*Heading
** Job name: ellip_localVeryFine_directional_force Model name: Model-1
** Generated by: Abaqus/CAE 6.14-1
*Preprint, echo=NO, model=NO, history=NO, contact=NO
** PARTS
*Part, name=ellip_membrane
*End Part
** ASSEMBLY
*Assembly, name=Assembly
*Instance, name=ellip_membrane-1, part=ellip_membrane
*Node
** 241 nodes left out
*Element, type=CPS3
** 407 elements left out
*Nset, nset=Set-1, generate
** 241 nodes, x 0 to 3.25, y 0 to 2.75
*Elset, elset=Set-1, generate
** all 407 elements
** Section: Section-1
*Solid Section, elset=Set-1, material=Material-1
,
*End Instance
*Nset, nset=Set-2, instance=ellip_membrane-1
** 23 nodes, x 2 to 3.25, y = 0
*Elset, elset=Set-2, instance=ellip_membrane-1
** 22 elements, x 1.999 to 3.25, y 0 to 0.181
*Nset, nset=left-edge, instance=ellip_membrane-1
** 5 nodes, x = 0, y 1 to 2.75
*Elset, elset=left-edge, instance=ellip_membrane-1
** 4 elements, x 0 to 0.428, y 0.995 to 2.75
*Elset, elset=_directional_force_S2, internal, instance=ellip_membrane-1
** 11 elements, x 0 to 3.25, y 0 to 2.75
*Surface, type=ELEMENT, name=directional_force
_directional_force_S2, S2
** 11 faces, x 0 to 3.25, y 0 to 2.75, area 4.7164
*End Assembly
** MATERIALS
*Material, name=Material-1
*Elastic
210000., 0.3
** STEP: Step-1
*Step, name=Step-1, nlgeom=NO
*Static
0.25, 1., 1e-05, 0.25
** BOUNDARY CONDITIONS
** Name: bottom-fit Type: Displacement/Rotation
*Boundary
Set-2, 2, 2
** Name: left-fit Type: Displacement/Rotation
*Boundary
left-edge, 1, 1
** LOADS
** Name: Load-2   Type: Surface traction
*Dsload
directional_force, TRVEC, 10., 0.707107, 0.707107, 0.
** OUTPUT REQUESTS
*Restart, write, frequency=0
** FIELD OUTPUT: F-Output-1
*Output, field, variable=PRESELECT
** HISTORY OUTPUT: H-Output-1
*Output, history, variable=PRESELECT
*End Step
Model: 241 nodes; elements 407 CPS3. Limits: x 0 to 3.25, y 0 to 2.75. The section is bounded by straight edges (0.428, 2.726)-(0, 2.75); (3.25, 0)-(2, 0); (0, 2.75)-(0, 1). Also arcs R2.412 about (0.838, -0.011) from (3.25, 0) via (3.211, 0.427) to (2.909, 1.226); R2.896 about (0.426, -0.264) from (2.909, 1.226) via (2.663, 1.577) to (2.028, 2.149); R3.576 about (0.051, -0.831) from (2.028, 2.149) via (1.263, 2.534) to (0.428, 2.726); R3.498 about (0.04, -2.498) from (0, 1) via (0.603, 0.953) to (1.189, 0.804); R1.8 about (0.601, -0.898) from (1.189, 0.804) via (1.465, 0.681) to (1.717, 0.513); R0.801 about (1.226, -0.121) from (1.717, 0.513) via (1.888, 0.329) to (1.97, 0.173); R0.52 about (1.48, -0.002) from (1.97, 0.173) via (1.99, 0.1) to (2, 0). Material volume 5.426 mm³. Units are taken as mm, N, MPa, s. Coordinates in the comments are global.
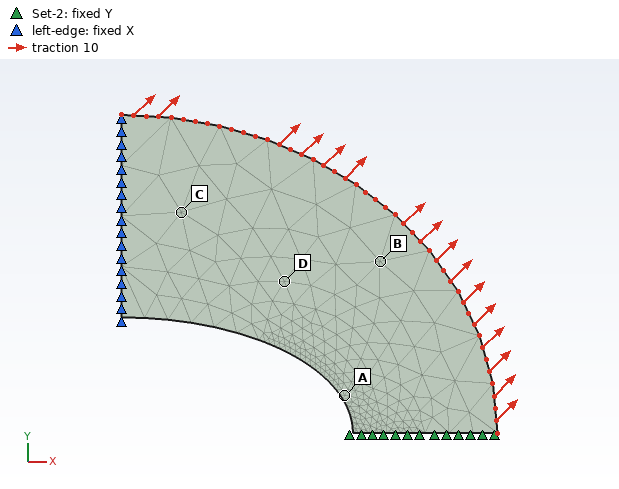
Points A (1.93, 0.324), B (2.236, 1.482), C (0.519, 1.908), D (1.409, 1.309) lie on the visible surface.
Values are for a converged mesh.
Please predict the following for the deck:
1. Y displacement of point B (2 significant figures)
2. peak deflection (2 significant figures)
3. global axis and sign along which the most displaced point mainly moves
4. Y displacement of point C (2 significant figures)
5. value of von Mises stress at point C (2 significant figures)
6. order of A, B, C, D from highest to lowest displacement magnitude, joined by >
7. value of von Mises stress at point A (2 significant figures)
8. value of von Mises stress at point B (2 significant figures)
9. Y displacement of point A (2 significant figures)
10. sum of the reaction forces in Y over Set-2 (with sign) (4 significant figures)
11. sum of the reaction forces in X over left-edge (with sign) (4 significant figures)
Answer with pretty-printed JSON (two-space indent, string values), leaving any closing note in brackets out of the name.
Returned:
{
  "Y displacement of point B": "1.6e-04 mm",
  "peak deflection": "4.7e-04 mm",
  "global axis and sign along which the most displaced point mainly moves": "+Y",
  "Y displacement of point C": "4.5e-04 mm",
  "value of von Mises stress at point C": "18 MPa",
  "order of A, B, C, D from highest to lowest displacement magnitude, joined by >": "C > D > B > A",
  "value of von Mises stress at point A": "50 MPa",
  "value of von Mises stress at point B": "13 MPa",
  "Y displacement of point A": "1.1e-04 mm",
  "sum of the reaction forces in Y over Set-2 (with sign)": "-33.35 N",
  "sum of the reaction forces in X over left-edge (with sign)": "-33.35 N"
}
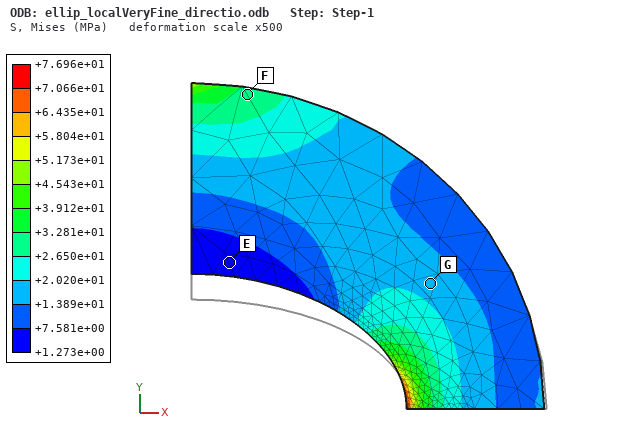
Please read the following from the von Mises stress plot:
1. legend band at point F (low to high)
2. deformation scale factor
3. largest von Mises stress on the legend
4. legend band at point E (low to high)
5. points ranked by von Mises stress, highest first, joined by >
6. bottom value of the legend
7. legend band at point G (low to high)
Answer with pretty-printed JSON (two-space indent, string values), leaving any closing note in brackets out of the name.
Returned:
{
  "legend band at point F": "+2.650e+01 to +3.281e+01 MPa",
  "deformation scale factor": "500",
  "largest von Mises stress on the legend": "+7.696e+01 MPa",
  "legend band at point E": "+1.273e+00 to +7.581e+00 MPa",
  "points ranked by von Mises stress, highest first, joined by >": "F > G > E",
  "bottom value of the legend": "+1.273e+00 MPa",
  "legend band at point G": "+1.389e+01 to +2.020e+01 MPa"
}
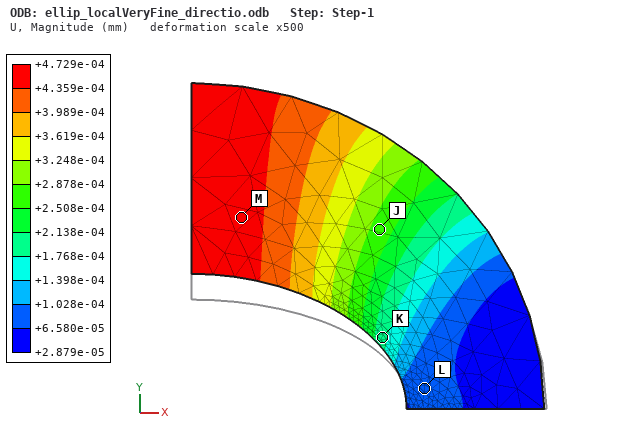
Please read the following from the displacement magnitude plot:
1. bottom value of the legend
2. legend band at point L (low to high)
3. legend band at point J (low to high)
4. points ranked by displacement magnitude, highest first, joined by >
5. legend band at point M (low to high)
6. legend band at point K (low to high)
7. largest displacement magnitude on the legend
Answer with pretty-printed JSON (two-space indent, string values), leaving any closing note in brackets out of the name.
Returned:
{
  "bottom value of the legend": "+2.879e-05 mm",
  "legend band at point L": "+6.580e-05 to +1.028e-04 mm",
  "legend band at point J": "+2.508e-04 to +2.878e-04 mm",
  "points ranked by displacement magnitude, highest first, joined by >": "M > J > K > L",
  "legend band at point M": "+4.359e-04 to +4.729e-04 mm",
  "legend band at point K": "+1.768e-04 to +2.138e-04 mm",
  "largest displacement magnitude on the legend": "+4.729e-04 mm"
}
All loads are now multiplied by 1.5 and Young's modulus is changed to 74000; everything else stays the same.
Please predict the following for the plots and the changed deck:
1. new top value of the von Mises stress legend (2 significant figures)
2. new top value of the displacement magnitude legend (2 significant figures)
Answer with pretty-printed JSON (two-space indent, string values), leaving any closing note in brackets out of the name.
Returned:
{
  "new top value of the von Mises stress legend": "120 MPa",
  "new top value of the displacement magnitude legend": "0.0020 mm"
}
